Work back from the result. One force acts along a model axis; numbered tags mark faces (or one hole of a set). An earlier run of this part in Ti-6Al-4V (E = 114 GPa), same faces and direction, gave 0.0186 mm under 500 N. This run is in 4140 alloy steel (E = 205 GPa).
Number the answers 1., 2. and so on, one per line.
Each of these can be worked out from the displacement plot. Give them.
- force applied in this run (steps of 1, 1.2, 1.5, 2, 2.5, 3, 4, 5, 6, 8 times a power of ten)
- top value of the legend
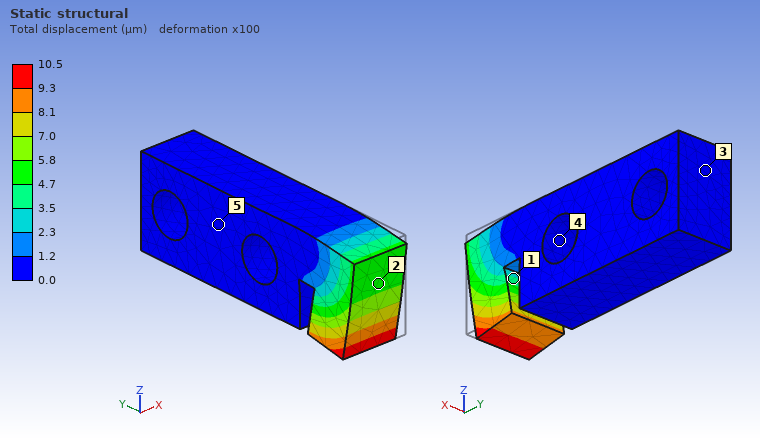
1. 500 N
2. 10.5 µm
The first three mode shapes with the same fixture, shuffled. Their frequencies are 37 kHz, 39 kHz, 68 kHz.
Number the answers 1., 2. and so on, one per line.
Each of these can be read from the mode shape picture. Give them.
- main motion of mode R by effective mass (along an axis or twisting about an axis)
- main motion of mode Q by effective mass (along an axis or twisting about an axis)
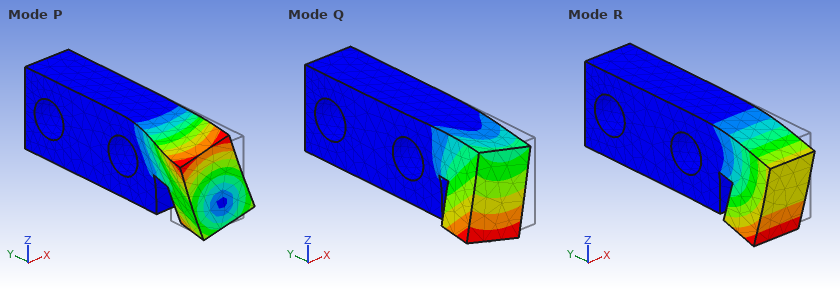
1. along Z
2. along X
